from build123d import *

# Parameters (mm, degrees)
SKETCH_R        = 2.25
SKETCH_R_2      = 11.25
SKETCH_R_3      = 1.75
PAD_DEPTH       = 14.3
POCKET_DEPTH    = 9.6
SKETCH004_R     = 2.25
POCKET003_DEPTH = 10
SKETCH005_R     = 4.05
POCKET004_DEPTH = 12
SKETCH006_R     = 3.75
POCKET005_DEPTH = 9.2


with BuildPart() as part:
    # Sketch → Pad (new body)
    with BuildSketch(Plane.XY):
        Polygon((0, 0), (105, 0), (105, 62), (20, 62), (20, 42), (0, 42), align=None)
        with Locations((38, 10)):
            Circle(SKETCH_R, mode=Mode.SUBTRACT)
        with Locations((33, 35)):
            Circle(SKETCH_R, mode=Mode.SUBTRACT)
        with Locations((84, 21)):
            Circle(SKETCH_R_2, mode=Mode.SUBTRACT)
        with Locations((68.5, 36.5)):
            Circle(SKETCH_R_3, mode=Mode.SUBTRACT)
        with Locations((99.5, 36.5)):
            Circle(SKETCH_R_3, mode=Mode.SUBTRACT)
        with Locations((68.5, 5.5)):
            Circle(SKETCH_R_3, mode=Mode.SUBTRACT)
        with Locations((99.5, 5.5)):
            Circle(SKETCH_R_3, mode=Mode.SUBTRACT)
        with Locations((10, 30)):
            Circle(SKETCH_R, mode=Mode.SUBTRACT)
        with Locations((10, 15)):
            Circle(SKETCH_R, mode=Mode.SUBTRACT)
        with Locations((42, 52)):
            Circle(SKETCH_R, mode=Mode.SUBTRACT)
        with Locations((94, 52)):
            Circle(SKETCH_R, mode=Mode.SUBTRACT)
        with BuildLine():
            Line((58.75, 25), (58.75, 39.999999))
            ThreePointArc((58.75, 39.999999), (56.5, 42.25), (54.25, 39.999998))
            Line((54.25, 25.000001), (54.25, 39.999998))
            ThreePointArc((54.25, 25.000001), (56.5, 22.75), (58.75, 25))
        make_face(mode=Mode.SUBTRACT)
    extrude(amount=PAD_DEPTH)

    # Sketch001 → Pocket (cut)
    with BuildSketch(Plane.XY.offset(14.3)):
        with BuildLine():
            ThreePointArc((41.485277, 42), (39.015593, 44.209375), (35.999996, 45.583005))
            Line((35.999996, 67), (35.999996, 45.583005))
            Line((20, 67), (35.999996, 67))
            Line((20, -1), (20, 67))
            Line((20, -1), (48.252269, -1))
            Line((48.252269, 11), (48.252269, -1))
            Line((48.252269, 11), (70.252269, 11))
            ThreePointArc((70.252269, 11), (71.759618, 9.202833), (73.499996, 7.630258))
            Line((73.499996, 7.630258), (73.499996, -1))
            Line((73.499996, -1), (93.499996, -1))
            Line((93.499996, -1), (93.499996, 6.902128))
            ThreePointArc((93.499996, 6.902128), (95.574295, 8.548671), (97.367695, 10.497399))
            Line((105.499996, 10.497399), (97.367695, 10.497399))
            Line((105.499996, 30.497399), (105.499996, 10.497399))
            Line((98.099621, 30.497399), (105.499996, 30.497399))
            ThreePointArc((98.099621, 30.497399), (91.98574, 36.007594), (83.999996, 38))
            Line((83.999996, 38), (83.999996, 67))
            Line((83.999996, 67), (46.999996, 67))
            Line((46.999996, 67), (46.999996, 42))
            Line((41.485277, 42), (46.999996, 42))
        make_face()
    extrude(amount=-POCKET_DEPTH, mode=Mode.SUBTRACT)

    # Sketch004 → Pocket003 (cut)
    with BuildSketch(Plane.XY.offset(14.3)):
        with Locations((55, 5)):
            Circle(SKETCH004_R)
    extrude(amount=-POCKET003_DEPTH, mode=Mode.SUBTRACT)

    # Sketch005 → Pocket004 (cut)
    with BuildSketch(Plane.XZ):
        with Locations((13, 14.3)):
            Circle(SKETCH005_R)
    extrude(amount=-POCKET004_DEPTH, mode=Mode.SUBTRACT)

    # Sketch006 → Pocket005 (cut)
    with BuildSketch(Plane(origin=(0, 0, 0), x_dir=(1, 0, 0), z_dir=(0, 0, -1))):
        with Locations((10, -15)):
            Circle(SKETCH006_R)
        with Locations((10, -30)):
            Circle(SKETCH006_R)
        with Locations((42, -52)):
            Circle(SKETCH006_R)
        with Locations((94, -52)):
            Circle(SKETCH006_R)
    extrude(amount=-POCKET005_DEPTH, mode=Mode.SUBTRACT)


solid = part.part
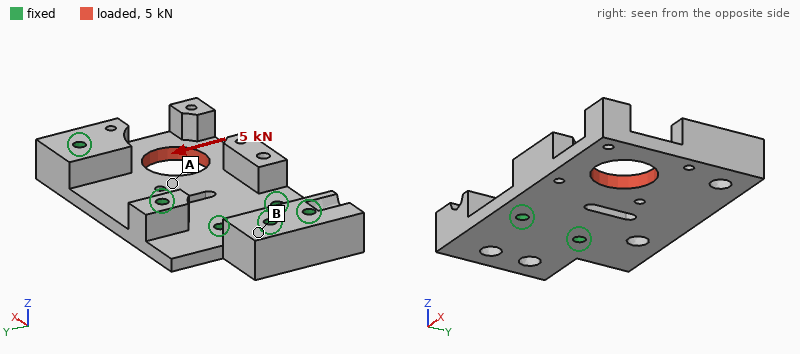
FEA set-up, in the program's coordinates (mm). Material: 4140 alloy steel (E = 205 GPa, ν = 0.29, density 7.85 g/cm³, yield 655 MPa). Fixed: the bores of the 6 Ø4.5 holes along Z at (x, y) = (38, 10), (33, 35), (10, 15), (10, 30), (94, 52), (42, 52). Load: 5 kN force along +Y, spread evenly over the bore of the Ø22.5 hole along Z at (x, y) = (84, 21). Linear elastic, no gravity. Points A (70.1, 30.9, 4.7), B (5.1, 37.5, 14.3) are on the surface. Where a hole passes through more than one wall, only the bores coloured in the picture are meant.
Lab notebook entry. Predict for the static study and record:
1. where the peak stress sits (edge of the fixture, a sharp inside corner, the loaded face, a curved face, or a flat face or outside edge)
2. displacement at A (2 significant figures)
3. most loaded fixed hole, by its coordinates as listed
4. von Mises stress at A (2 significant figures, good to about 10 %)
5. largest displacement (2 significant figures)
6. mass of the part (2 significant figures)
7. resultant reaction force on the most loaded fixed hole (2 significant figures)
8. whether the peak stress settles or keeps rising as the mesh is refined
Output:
edge of the fixture
13 µm
(94, 52)
28 MPa
45 µm
340 g
2.7 kN
keeps rising
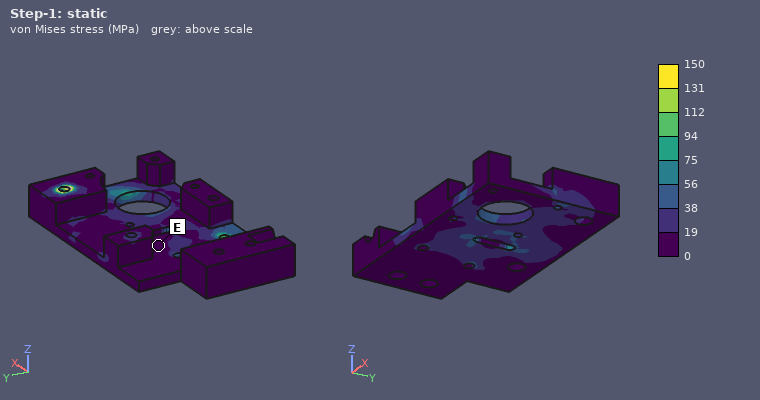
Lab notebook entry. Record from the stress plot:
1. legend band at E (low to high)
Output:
0 to 19 MPa
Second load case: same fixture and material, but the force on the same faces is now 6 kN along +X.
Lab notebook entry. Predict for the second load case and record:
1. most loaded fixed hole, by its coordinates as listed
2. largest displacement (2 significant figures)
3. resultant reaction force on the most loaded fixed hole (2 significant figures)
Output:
(38, 10)
14 µm
2.9 kN
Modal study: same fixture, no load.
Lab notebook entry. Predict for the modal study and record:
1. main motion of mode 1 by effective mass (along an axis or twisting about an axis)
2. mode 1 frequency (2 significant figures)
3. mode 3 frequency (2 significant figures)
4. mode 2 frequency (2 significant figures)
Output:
along Z
2300 Hz
6500 Hz
5100 Hz
